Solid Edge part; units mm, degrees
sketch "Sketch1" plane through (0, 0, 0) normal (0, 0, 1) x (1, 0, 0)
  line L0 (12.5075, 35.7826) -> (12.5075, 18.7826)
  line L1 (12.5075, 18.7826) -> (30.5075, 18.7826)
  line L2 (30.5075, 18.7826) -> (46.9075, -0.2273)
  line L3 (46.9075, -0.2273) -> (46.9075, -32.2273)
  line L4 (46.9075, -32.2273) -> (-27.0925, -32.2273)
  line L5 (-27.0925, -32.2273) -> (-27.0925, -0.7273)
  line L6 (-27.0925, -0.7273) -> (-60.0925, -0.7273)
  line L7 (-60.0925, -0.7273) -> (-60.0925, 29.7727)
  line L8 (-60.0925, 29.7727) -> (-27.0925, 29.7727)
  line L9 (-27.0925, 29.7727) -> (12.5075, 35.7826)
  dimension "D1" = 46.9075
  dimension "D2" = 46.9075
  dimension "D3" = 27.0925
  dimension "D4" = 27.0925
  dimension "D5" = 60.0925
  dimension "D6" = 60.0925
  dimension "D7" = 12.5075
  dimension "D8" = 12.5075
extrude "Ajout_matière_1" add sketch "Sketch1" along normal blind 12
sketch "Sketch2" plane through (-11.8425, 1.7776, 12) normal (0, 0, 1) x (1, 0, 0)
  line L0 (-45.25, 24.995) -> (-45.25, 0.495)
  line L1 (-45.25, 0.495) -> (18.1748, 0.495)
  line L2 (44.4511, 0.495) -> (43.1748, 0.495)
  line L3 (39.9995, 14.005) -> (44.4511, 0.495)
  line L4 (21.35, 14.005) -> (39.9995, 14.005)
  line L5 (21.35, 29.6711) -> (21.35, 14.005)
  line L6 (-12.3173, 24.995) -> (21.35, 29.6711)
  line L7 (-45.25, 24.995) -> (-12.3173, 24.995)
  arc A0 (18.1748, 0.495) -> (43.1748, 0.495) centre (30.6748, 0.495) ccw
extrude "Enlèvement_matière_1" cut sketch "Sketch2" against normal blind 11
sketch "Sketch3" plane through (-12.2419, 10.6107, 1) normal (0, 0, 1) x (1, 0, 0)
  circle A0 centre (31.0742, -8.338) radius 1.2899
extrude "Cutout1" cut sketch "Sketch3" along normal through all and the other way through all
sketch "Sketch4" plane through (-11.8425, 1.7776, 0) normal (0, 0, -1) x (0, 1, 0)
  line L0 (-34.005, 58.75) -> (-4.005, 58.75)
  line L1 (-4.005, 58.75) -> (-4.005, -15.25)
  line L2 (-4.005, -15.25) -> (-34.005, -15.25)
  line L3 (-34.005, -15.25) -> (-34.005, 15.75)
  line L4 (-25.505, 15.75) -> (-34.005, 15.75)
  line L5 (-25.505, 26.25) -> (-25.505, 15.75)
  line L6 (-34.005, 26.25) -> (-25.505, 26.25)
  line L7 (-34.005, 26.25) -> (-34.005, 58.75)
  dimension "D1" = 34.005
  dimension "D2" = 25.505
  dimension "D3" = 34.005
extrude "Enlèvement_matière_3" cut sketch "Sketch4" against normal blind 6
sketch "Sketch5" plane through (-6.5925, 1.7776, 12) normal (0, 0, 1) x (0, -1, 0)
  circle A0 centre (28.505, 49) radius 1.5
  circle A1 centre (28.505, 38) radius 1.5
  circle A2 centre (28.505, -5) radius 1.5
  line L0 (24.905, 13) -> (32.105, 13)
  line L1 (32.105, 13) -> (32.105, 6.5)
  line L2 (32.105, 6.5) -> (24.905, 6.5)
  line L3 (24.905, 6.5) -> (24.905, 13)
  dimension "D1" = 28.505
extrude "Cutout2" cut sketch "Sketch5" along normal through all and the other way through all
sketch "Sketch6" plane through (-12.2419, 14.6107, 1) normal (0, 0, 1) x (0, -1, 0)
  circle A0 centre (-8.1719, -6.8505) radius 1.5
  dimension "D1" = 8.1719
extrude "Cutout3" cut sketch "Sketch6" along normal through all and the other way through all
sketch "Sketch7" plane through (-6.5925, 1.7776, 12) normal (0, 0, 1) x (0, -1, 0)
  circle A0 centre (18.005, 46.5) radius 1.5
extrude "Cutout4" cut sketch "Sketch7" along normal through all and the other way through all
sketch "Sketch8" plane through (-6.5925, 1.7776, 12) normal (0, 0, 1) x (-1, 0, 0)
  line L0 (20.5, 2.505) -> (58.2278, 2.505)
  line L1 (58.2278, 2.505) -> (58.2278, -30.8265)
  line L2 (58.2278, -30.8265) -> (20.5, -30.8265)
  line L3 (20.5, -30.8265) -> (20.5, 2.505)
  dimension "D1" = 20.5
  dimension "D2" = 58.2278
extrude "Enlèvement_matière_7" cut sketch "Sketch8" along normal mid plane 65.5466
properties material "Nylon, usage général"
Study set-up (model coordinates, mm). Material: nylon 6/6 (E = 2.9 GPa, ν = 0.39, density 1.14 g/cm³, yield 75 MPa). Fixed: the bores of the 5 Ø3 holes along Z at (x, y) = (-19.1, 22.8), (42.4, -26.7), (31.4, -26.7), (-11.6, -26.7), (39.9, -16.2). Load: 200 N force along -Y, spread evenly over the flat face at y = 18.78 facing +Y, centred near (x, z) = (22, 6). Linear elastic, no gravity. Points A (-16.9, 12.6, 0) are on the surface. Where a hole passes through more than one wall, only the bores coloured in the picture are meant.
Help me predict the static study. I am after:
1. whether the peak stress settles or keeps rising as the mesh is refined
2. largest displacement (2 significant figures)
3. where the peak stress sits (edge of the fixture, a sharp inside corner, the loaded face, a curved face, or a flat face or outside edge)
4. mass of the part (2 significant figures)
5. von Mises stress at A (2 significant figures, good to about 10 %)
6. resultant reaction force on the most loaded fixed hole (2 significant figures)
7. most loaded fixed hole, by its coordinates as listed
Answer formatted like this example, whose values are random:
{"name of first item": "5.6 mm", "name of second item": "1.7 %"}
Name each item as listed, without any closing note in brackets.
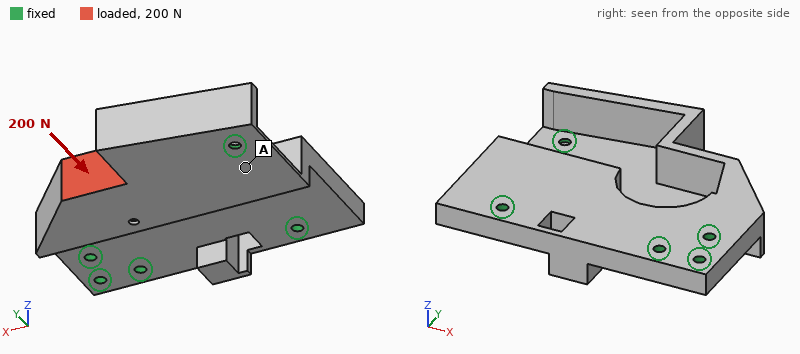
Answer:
{"whether the peak stress settles or keeps rising as the mesh is refined": "keeps rising", "largest displacement": "0.79 mm", "where the peak stress sits": "edge of the fixture", "mass of the part": "24 g", "von Mises stress at A": "2.8 MPa", "resultant reaction force on the most loaded fixed hole": "86 N", "most loaded fixed hole, by its coordinates as listed": "(39.9, -16.2)"}
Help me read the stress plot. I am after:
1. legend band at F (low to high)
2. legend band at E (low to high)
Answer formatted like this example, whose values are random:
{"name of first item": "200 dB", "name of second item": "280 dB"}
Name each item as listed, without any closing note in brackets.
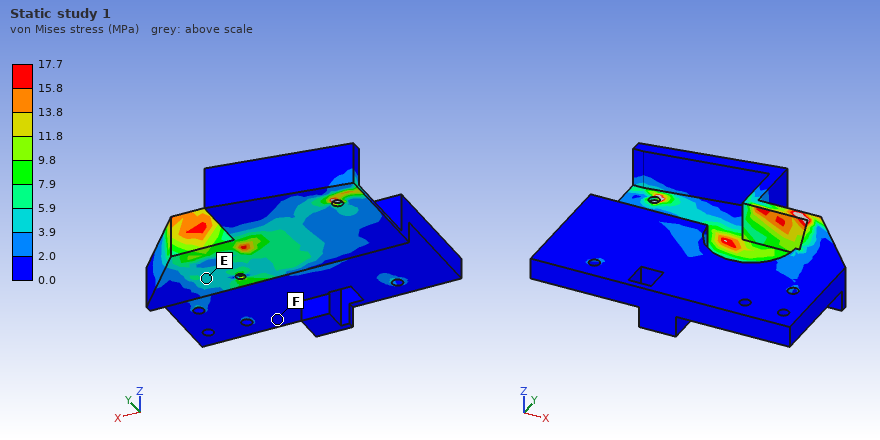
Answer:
{"legend band at F": "0.0 to 2.0 MPa", "legend band at E": "3.9 to 5.9 MPa"}
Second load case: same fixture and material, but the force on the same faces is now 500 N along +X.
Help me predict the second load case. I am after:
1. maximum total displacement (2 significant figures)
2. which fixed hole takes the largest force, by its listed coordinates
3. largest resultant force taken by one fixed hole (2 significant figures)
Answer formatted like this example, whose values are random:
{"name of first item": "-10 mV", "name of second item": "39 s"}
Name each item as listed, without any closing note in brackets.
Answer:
{"maximum total displacement": "0.94 mm", "which fixed hole takes the largest force, by its listed coordinates": "(39.9, -16.2)", "largest resultant force taken by one fixed hole": "290 N"}
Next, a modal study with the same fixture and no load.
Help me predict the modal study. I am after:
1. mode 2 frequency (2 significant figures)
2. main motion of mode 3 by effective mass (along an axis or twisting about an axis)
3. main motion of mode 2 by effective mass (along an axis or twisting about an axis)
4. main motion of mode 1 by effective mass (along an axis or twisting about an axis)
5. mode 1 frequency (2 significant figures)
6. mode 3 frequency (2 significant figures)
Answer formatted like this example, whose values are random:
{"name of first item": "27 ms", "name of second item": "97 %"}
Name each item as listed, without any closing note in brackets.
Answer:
{"mode 2 frequency": "1300 Hz", "main motion of mode 3 by effective mass": "along Z", "main motion of mode 2 by effective mass": "along Z", "main motion of mode 1 by effective mass": "along Z", "mode 1 frequency": "650 Hz", "mode 3 frequency": "1700 Hz"}
